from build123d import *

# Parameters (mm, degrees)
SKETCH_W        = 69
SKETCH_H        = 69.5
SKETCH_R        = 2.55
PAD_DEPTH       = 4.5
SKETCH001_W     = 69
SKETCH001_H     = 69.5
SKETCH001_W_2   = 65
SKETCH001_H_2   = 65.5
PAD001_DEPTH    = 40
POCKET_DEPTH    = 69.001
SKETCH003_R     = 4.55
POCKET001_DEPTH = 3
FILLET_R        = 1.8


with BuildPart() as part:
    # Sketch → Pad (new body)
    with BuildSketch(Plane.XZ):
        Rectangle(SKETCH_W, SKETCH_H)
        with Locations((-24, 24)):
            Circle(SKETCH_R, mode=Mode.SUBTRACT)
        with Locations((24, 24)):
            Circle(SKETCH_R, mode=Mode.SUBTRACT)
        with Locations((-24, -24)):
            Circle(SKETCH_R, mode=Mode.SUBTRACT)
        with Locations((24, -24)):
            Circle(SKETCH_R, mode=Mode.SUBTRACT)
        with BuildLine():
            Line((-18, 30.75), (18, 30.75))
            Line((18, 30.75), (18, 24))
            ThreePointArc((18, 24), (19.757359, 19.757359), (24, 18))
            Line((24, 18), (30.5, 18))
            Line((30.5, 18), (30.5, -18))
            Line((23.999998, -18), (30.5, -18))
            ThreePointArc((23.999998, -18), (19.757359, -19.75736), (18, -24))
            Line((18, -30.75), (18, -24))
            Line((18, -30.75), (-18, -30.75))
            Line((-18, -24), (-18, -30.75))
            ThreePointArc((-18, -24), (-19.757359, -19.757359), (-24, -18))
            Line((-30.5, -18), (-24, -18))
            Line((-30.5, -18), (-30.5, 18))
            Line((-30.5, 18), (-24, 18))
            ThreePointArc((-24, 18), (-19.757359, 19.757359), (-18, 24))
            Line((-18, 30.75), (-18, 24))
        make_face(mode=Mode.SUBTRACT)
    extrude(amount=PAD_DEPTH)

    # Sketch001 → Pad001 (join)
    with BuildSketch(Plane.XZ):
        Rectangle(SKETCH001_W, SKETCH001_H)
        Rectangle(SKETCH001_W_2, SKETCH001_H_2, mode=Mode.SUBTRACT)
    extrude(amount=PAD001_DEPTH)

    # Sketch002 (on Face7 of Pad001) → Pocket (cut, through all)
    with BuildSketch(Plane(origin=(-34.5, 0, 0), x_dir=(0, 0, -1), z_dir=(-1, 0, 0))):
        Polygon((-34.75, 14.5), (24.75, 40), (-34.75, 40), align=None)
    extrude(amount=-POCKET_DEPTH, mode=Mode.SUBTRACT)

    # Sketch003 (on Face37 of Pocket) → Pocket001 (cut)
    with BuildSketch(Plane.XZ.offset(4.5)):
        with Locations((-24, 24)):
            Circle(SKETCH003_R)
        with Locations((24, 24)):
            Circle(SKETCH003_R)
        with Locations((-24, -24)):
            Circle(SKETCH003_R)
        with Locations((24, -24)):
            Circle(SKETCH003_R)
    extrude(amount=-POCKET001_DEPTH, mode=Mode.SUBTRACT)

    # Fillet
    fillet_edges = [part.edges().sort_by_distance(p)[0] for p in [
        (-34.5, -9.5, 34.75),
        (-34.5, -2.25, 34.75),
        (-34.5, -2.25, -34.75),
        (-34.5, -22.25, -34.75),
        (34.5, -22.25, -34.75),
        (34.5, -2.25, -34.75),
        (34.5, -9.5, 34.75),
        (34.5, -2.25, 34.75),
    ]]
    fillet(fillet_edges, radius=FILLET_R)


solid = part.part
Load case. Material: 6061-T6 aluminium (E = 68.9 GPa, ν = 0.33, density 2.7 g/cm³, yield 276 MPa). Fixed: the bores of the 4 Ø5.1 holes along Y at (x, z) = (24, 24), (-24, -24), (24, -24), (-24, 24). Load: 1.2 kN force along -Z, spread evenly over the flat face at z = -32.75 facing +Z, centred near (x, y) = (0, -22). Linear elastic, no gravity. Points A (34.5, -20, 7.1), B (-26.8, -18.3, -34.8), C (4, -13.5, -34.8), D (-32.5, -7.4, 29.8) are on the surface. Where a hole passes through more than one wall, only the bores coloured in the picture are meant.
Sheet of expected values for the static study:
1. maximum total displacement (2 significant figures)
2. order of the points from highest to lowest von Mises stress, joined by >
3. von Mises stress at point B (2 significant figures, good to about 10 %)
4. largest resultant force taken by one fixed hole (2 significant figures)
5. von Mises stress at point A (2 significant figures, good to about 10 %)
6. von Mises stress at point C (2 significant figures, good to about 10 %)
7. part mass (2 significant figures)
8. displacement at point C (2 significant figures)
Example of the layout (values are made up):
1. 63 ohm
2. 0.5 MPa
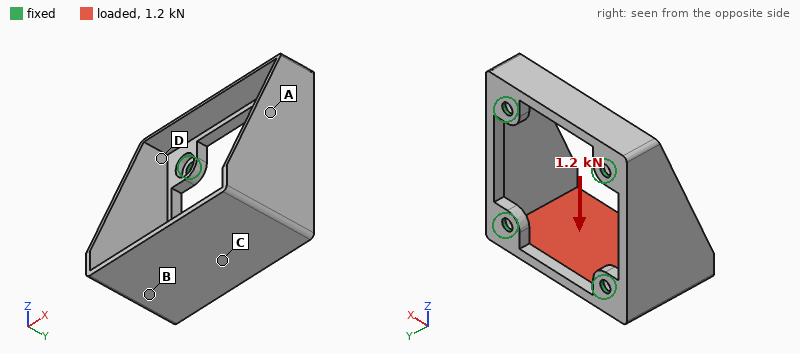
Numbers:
1. 0.89 mm
2. B > C > A > D
3. 99 MPa
4. 620 N
5. 27 MPa
6. 63 MPa
7. 52 g
8. 0.26 mm
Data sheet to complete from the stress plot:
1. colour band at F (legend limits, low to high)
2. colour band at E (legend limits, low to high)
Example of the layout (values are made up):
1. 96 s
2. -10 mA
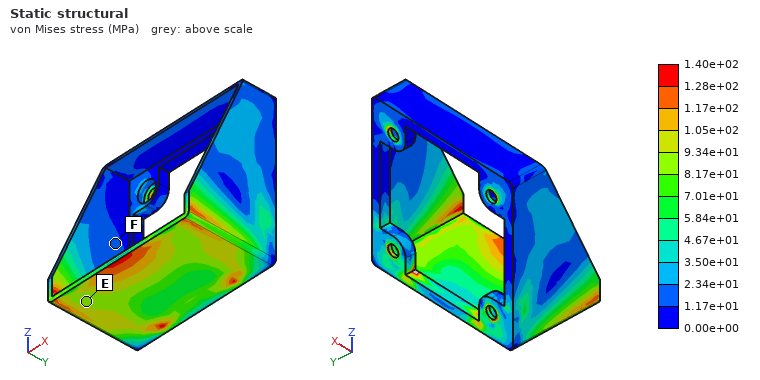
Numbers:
1. 1.17e+01 to 2.34e+01 MPa
2. 8.17e+01 to 9.34e+01 MPa
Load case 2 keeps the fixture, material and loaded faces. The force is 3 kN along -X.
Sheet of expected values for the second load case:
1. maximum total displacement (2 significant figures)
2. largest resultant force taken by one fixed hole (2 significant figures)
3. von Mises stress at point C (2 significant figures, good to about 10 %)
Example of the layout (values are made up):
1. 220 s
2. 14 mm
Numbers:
1. 0.20 mm
2. 2.0 kN
3. 44 MPa
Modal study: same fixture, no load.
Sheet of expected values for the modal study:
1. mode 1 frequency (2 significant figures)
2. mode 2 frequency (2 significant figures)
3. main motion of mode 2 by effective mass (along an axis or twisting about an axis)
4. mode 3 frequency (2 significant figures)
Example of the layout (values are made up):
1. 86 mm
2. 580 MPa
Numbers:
1. 2100 Hz
2. 2700 Hz
3. along X
4. 3100 Hz
